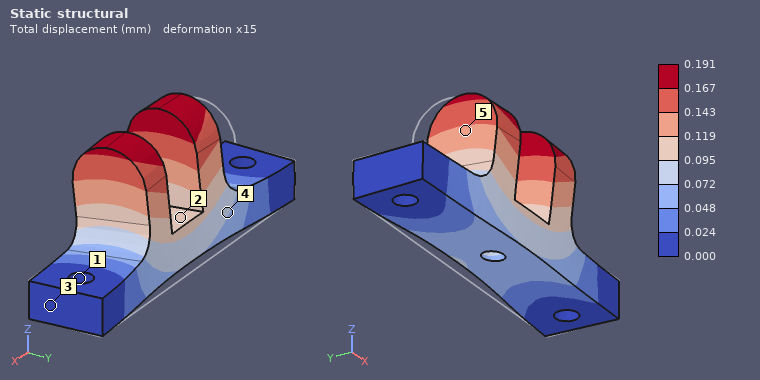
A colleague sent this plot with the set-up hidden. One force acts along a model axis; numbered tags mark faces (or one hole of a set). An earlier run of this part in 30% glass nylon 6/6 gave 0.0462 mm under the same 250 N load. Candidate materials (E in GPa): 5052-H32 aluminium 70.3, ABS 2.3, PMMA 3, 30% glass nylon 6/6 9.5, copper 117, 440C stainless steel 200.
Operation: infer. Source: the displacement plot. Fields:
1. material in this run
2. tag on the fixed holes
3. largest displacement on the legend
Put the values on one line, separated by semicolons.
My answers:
ABS; 1; 0.191 mm
